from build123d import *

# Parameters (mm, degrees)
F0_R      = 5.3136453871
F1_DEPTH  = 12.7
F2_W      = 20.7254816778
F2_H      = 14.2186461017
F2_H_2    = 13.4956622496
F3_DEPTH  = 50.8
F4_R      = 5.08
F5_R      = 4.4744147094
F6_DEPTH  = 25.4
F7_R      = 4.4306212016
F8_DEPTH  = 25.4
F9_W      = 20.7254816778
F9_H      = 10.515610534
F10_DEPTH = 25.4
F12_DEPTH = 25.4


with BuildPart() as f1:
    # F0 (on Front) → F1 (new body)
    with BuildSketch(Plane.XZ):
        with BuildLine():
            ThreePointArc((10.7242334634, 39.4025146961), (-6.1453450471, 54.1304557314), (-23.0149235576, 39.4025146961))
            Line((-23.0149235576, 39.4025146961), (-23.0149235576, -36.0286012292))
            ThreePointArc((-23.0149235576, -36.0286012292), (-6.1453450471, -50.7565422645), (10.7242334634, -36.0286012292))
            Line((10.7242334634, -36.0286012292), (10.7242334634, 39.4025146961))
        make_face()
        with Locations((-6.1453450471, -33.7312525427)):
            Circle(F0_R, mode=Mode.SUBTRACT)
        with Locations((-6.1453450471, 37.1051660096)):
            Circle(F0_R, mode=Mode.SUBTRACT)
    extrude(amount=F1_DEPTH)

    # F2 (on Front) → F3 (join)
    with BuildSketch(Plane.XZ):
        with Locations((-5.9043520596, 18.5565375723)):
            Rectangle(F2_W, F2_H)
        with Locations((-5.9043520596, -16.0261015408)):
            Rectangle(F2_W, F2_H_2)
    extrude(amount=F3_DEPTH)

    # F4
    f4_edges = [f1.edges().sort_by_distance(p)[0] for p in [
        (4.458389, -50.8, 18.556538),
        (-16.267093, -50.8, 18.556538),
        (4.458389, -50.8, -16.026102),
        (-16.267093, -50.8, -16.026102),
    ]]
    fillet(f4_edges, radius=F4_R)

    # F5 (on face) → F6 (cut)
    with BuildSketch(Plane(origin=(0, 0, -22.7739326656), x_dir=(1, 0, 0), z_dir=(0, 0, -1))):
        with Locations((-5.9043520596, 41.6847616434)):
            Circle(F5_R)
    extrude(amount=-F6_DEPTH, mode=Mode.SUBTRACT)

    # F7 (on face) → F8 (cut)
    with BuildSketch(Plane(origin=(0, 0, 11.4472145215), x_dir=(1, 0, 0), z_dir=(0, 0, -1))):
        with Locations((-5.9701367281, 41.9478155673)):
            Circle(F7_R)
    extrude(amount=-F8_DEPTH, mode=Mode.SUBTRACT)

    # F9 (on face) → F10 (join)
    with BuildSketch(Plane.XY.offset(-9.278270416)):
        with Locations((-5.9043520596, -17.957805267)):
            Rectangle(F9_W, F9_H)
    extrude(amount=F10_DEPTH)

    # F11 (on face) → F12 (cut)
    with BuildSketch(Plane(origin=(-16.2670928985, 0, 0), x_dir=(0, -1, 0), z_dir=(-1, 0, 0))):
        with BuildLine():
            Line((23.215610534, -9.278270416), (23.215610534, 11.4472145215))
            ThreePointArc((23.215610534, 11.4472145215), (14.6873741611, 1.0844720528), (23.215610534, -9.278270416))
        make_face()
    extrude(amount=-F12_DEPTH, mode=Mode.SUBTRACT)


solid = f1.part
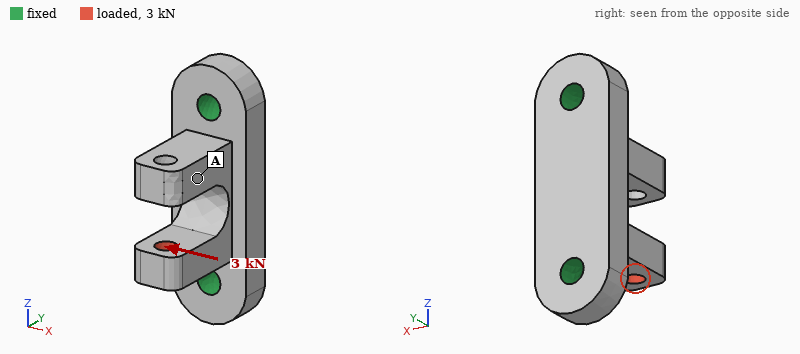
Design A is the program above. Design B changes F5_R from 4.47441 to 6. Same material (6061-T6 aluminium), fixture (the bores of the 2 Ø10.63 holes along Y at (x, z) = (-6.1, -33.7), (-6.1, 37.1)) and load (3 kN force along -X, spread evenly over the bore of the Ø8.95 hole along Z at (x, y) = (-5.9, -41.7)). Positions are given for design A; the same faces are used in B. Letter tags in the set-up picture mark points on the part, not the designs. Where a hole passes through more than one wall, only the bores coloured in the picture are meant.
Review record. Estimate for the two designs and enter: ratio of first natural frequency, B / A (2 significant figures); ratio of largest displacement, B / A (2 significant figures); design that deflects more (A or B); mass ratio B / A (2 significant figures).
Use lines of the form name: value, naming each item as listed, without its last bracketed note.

ratio of first natural frequency, B / A: 1.0
ratio of largest displacement, B / A: 1.1
design that deflects more: B
mass ratio B / A: 0.99
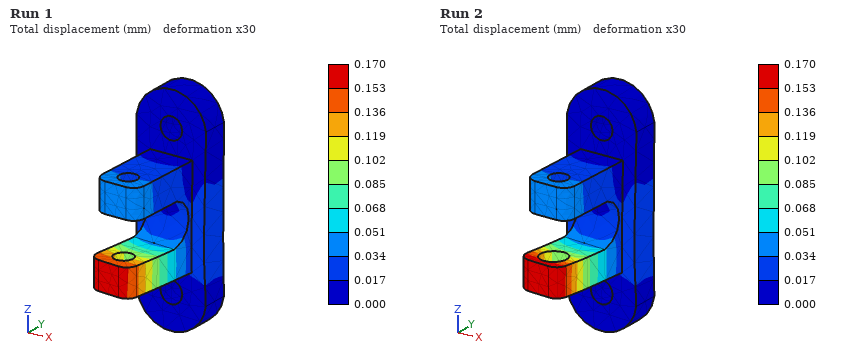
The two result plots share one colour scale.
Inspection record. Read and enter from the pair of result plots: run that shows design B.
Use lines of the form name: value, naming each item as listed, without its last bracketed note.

run that shows design B: Run 2
